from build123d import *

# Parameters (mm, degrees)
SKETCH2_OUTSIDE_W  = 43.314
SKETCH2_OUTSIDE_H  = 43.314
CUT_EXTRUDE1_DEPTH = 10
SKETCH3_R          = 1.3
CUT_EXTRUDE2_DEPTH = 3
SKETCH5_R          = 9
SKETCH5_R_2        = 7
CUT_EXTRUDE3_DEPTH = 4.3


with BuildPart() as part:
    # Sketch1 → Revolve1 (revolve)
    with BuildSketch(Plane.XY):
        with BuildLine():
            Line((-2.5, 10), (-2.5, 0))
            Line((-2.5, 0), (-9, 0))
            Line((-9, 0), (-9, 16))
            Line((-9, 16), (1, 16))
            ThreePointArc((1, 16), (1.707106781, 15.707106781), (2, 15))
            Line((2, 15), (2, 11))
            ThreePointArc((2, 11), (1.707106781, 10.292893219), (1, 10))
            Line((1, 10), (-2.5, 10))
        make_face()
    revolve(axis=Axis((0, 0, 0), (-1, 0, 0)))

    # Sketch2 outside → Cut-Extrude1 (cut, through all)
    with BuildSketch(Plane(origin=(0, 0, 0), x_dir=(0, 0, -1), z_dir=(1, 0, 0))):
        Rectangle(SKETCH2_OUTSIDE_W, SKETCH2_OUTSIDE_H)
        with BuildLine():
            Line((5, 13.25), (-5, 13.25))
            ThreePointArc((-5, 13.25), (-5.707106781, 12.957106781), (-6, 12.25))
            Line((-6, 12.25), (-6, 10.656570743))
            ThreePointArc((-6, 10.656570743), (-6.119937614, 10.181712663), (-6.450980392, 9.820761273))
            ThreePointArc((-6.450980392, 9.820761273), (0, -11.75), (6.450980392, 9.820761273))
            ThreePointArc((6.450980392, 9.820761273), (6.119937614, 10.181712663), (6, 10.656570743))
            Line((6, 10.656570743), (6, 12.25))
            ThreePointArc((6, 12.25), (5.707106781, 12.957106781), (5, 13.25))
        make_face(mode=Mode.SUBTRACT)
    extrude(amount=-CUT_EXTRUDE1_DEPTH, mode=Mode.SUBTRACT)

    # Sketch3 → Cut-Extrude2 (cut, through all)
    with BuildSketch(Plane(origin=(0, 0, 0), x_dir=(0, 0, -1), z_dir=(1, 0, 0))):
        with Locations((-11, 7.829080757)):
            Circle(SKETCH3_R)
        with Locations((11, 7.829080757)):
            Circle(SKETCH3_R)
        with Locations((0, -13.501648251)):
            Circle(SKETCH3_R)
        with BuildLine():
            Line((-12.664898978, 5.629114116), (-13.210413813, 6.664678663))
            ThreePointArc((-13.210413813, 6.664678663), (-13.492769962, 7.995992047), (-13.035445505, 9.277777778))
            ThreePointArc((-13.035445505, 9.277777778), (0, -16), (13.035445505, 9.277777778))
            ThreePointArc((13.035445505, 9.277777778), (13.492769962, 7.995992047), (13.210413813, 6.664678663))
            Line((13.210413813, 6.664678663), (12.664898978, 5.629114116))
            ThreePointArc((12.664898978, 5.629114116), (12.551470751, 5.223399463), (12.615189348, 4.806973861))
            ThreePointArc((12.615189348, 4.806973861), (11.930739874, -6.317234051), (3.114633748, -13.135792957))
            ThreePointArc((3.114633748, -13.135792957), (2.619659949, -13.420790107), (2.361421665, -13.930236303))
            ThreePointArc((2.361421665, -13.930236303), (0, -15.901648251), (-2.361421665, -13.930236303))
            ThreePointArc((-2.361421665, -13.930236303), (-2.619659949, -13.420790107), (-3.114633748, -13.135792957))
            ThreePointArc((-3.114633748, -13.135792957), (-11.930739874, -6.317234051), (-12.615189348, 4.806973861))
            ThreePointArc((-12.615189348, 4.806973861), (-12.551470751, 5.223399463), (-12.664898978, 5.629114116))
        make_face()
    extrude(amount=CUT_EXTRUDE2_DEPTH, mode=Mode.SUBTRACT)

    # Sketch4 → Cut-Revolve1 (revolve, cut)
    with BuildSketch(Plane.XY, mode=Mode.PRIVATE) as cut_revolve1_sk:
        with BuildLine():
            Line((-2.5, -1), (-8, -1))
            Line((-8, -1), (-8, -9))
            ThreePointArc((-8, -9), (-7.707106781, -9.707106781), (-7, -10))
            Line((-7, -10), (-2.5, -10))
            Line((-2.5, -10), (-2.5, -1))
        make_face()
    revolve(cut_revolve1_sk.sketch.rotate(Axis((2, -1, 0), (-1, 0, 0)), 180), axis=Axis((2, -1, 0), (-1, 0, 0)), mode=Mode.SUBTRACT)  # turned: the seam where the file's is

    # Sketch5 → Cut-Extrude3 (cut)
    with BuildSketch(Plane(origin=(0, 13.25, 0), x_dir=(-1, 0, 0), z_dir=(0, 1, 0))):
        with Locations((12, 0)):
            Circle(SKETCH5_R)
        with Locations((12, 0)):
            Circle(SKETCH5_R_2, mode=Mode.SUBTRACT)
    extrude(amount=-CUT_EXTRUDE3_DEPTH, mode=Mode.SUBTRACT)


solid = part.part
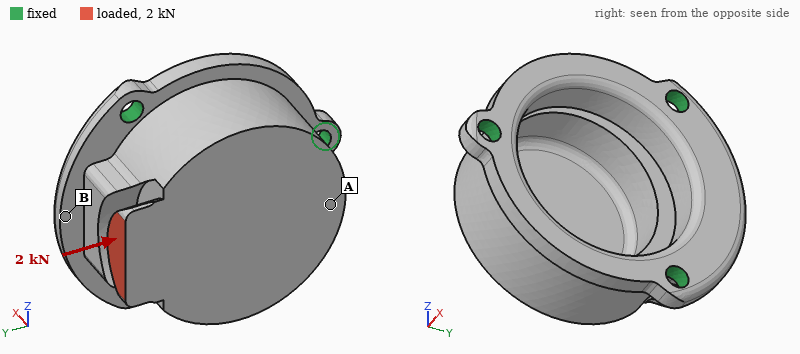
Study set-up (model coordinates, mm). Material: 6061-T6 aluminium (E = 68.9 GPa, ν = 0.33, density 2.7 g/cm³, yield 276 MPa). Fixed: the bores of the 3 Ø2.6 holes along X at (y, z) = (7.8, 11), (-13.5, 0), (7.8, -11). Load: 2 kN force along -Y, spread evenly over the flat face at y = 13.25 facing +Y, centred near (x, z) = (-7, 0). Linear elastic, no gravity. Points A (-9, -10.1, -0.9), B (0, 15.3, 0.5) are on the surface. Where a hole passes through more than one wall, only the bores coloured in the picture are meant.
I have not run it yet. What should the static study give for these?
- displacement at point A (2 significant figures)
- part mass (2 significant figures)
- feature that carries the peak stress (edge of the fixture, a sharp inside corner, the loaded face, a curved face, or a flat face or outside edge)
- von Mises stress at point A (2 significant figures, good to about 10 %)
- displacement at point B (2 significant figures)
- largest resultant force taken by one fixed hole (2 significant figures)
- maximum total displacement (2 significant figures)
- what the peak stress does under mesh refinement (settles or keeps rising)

24 µm
6.7 g
edge of the fixture
71 MPa
31 µm
960 N
41 µm
keeps rising
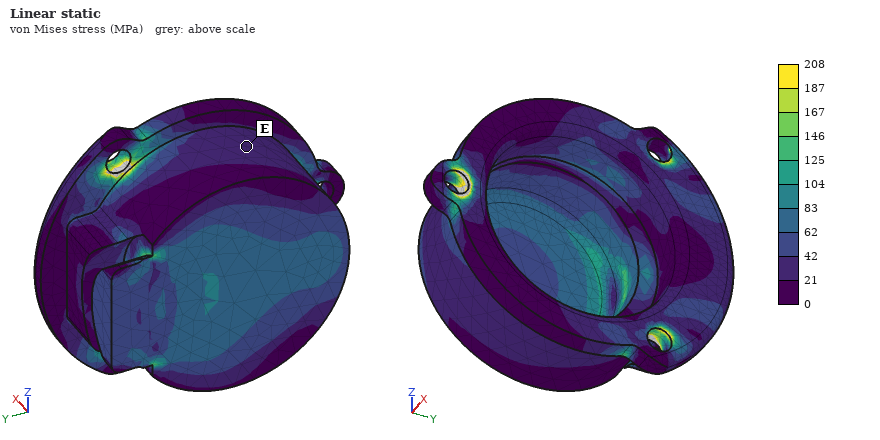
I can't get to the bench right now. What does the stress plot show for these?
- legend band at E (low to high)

21 to 42 MPa
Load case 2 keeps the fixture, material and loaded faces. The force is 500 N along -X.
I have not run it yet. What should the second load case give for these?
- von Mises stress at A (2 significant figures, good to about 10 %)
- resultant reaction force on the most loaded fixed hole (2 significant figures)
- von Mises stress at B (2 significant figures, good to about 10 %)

16 MPa
430 N
11 MPa
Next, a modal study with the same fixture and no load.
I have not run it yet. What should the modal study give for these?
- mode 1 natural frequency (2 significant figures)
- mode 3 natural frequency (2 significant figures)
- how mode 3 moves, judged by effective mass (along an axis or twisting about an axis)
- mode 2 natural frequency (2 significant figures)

21 kHz
26 kHz
along X
21 kHz
